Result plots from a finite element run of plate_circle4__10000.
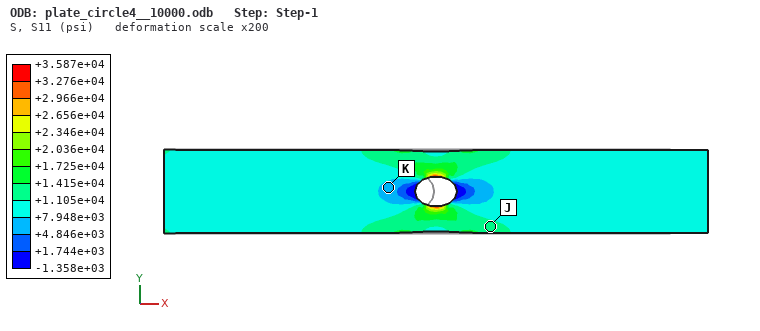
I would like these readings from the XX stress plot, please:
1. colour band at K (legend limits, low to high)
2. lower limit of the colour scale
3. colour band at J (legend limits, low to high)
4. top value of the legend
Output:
+4.846e+03 to +7.948e+03 psi
-1.358e+03 psi
+1.105e+04 to +1.415e+04 psi
+3.587e+04 psi
